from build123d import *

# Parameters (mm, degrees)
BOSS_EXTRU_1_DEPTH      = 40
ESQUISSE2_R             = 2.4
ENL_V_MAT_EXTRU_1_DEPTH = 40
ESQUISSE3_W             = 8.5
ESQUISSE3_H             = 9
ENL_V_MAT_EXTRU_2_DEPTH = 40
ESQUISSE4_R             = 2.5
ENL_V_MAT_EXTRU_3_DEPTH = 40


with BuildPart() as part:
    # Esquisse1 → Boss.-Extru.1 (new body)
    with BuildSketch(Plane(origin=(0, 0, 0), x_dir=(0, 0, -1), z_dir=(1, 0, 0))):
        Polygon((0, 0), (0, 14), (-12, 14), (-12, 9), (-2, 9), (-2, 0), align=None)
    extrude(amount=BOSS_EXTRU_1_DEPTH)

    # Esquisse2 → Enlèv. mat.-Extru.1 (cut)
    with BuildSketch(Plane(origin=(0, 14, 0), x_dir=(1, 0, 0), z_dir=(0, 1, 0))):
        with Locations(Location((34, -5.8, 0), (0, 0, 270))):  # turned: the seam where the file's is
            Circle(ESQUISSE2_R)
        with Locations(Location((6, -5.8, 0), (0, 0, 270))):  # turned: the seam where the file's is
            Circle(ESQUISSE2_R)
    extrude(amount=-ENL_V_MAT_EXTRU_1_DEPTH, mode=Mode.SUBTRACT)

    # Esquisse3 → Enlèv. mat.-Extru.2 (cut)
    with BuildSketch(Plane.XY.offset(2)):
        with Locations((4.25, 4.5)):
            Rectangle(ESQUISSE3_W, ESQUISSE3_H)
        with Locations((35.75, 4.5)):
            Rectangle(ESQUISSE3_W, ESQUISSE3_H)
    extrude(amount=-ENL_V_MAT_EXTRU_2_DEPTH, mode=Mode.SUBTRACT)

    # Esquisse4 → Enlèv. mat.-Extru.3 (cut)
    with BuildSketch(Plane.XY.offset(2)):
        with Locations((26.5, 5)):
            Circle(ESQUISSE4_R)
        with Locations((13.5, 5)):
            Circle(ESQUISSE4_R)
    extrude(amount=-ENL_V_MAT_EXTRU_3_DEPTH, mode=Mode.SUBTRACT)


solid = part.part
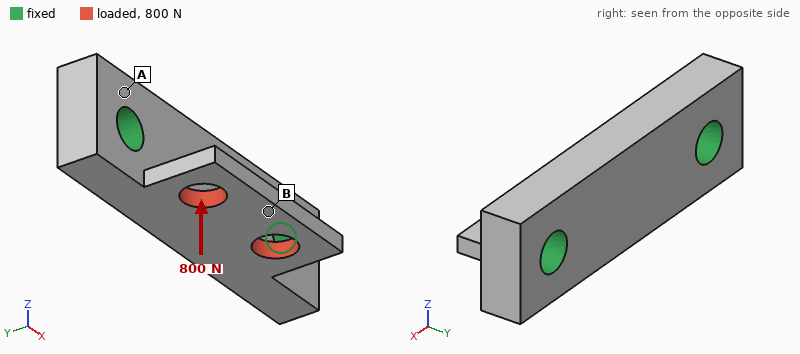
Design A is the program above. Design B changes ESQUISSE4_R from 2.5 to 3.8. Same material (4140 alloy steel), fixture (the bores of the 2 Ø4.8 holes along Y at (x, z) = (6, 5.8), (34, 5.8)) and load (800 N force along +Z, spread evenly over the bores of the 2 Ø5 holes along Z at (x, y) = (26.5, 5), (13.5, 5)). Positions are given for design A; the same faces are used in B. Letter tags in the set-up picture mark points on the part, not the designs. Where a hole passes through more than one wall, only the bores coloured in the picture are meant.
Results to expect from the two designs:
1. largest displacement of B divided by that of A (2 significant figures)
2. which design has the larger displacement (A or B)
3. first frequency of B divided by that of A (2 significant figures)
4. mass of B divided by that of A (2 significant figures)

1.7
B
0.91
0.96
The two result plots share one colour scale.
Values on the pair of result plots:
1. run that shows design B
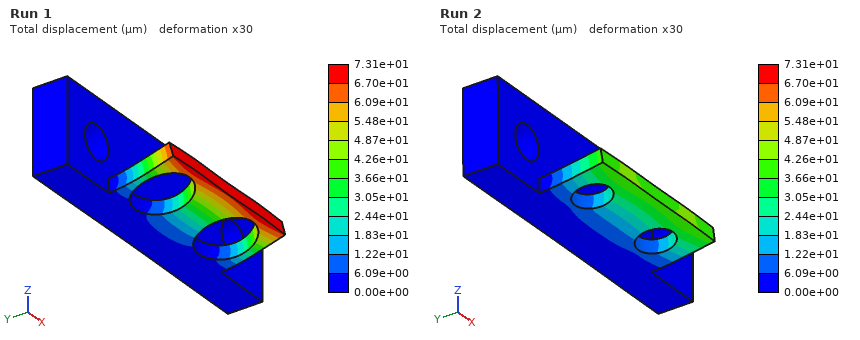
Run 1
